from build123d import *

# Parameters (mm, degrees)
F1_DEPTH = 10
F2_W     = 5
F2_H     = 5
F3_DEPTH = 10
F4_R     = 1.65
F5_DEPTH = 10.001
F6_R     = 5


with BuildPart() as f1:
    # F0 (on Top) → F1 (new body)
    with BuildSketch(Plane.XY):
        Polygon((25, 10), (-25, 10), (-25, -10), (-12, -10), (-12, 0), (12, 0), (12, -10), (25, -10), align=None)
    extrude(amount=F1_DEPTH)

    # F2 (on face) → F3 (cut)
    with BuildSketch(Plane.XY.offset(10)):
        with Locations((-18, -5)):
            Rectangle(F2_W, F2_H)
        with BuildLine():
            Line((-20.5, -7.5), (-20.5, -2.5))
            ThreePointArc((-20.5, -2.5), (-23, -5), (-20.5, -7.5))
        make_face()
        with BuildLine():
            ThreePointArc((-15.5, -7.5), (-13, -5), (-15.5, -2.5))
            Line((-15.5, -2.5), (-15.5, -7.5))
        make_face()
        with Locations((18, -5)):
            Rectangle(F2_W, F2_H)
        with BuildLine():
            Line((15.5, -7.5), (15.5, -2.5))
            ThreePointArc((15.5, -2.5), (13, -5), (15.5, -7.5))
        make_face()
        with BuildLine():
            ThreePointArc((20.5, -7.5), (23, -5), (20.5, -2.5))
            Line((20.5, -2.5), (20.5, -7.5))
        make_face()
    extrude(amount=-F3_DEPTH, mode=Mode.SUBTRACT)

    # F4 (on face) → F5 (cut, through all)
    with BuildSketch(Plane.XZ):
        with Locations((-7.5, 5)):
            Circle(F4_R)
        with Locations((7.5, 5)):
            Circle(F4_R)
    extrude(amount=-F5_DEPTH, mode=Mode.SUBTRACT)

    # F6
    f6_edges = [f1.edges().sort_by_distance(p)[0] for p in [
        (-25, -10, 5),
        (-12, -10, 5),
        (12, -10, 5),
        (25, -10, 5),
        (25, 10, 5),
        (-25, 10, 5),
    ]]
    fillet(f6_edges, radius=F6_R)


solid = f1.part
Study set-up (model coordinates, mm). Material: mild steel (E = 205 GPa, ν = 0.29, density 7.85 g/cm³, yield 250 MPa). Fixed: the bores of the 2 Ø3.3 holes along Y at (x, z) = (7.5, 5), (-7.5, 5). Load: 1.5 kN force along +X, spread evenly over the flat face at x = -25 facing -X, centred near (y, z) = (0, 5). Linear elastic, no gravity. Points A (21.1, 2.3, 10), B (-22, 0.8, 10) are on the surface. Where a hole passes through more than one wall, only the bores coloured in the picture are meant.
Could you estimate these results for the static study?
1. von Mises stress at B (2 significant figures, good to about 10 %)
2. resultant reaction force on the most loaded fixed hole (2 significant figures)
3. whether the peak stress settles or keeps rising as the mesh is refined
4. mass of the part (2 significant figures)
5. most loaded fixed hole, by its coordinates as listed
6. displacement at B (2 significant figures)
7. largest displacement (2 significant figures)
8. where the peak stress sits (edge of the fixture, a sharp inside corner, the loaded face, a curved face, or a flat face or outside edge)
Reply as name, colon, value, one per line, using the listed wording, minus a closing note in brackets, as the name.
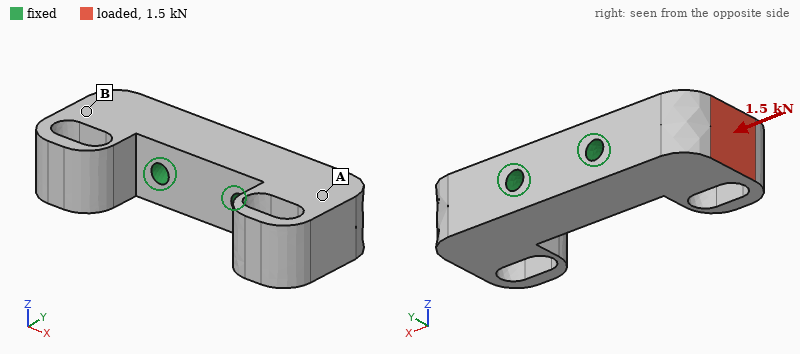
von Mises stress at B: 17 MPa
resultant reaction force on the most loaded fixed hole: 1.4 kN
whether the peak stress settles or keeps rising as the mesh is refined: keeps rising
mass of the part: 49 g
most loaded fixed hole, by its coordinates as listed: (-7.5, 5)
displacement at B: 4.7 µm
largest displacement: 8.8 µm
where the peak stress sits: edge of the fixture
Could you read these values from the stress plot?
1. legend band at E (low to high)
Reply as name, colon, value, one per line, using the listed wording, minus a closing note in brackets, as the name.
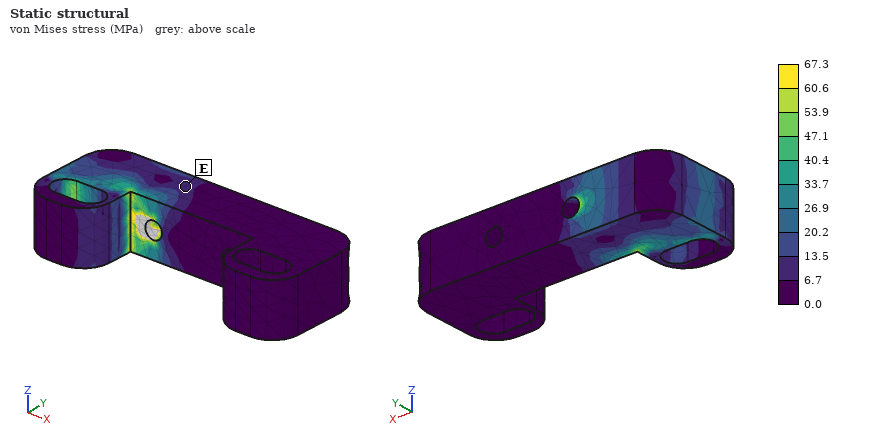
legend band at E: 6.7 to 13.5 MPa
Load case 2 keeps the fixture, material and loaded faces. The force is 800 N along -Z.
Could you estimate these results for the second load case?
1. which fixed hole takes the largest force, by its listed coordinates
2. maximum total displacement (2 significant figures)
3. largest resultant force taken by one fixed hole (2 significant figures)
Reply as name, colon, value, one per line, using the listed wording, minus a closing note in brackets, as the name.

which fixed hole takes the largest force, by its listed coordinates: (-7.5, 5)
maximum total displacement: 18 µm
largest resultant force taken by one fixed hole: 1.2 kN
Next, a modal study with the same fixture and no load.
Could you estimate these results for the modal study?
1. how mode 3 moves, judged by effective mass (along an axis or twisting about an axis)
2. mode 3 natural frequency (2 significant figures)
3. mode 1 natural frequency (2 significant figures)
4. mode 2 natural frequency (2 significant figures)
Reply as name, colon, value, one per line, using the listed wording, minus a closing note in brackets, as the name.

how mode 3 moves, judged by effective mass: along Y
mode 3 natural frequency: 15 kHz
mode 1 natural frequency: 14 kHz
mode 2 natural frequency: 14 kHz
